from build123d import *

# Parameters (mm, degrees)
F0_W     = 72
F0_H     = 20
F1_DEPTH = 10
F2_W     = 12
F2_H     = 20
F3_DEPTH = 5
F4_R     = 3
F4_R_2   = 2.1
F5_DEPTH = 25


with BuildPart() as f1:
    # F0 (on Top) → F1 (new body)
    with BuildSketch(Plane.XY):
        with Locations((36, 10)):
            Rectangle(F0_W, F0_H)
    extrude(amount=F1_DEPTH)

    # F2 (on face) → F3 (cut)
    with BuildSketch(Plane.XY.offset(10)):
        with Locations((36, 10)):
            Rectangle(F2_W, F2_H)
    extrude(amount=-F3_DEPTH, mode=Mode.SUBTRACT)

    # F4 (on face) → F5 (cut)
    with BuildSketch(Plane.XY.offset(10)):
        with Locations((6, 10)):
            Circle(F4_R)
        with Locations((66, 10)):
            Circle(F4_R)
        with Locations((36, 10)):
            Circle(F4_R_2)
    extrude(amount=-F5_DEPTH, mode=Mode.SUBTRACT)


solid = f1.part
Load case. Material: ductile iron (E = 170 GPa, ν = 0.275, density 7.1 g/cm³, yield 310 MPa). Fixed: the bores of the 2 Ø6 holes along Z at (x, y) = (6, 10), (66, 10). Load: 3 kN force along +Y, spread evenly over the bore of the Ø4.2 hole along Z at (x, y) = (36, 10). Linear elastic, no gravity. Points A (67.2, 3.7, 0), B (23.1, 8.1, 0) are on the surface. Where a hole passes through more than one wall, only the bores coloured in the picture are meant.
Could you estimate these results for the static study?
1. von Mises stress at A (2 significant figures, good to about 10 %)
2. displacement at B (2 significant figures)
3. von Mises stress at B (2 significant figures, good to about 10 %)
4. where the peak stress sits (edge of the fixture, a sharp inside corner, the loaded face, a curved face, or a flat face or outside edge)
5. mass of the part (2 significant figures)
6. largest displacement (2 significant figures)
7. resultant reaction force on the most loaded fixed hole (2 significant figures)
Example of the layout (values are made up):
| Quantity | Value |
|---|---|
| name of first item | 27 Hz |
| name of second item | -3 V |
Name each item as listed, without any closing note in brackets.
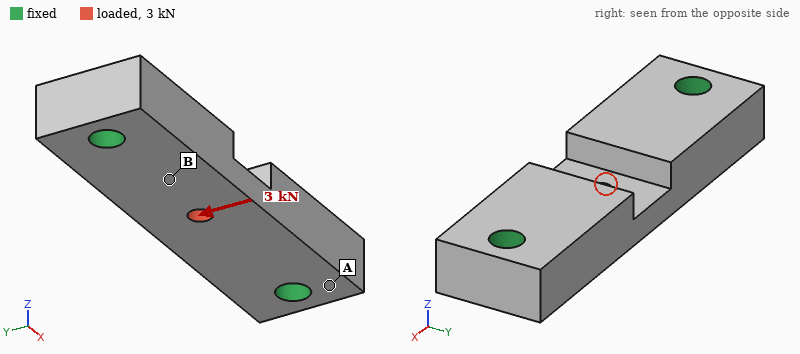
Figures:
| Quantity | Value |
|---|---|
| von Mises stress at A | 15 MPa |
| displacement at B | 8.2 µm |
| von Mises stress at B | 38 MPa |
| where the peak stress sits | edge of the fixture |
| mass of the part | 89 g |
| largest displacement | 14 µm |
| resultant reaction force on the most loaded fixed hole | 1.5 kN |
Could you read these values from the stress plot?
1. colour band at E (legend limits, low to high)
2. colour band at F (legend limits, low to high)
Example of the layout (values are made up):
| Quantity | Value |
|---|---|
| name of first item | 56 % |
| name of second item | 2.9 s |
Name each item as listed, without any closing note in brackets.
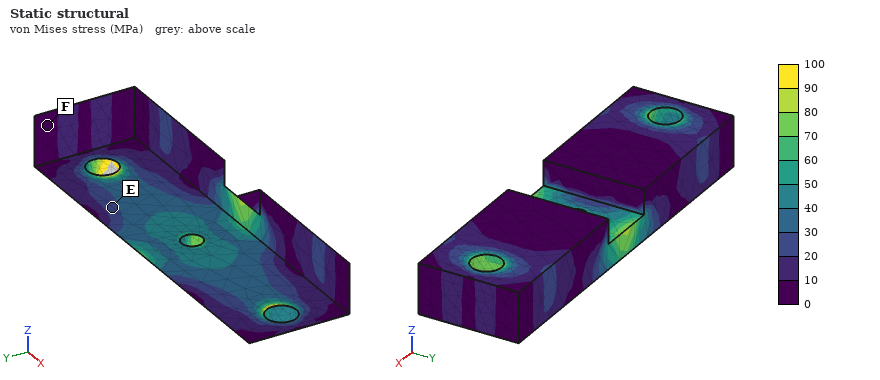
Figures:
| Quantity | Value |
|---|---|
| colour band at E | 20 to 30 MPa |
| colour band at F | 0 to 10 MPa |
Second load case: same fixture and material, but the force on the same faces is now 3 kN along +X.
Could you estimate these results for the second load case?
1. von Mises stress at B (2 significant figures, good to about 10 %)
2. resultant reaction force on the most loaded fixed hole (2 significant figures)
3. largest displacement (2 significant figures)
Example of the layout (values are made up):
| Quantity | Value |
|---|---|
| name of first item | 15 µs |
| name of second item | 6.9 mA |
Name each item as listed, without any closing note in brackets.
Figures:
| Quantity | Value |
|---|---|
| von Mises stress at B | 16 MPa |
| resultant reaction force on the most loaded fixed hole | 1.5 kN |
| largest displacement | 2.8 µm |
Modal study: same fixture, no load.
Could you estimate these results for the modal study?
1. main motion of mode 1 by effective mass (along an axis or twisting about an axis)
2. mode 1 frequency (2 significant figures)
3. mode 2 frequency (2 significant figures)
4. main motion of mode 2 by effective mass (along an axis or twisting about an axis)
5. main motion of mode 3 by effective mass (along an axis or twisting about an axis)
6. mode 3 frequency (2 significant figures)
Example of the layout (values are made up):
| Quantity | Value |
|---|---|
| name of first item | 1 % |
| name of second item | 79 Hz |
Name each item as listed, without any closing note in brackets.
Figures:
| Quantity | Value |
|---|---|
| main motion of mode 1 by effective mass | along Z |
| mode 1 frequency | 12 kHz |
| mode 2 frequency | 15 kHz |
| main motion of mode 2 by effective mass | along Y |
| main motion of mode 3 by effective mass | twisting about X |
| mode 3 frequency | 22 kHz |
